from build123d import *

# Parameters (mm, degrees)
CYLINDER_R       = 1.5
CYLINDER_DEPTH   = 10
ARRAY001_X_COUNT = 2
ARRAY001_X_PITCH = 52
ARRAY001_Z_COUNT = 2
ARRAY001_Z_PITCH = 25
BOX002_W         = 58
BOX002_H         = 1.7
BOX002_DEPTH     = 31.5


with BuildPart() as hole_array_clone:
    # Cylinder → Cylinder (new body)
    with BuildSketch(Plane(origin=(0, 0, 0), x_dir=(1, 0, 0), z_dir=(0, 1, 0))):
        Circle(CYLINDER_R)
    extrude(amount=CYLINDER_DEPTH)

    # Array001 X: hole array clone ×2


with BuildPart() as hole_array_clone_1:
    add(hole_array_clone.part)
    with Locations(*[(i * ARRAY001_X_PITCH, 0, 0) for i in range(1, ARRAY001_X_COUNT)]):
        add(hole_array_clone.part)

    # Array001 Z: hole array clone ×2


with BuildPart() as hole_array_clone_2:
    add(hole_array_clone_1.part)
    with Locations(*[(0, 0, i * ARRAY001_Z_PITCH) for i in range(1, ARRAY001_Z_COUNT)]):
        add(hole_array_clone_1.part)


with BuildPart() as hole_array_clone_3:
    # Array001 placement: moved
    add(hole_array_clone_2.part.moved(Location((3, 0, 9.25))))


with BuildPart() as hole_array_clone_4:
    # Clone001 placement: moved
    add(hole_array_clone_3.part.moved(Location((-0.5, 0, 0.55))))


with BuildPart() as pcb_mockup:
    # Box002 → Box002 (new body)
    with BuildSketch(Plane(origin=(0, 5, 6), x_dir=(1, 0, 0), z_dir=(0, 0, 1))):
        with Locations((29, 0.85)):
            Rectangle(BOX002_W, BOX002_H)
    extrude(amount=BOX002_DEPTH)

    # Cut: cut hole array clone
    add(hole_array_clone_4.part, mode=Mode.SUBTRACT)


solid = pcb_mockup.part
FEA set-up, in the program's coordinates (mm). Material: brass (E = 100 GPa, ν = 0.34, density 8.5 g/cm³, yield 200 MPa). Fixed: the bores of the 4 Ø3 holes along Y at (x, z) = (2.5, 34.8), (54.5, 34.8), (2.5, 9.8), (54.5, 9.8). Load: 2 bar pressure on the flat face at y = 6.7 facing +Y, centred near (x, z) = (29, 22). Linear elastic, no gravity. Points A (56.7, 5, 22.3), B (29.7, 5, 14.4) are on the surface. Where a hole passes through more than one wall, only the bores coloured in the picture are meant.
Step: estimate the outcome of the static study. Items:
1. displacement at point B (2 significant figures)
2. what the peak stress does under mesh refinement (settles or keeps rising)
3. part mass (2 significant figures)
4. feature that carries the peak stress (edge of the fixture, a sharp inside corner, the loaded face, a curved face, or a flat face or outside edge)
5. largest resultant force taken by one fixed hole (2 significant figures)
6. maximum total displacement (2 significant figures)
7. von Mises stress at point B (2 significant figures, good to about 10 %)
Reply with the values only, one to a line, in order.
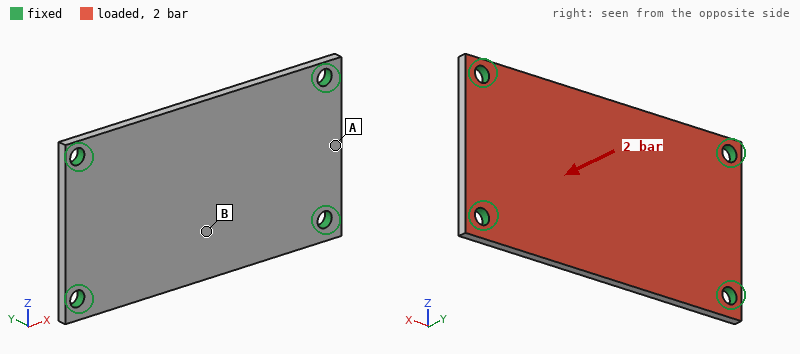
0.100 mm
keeps rising
26 g
edge of the fixture
95 N
0.11 mm
45 MPa
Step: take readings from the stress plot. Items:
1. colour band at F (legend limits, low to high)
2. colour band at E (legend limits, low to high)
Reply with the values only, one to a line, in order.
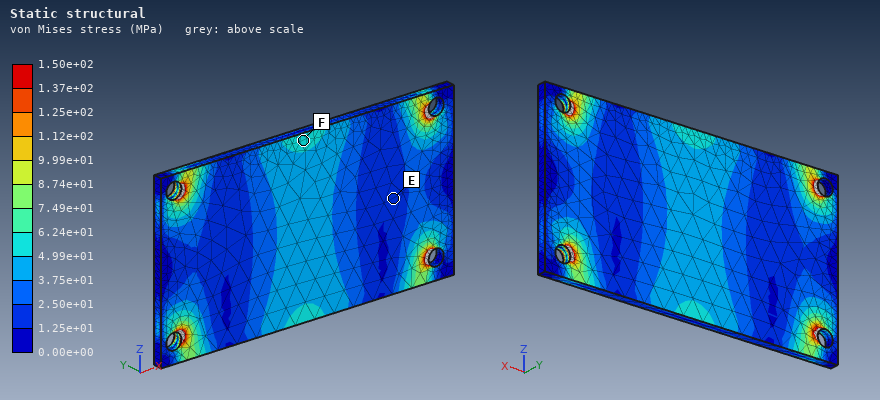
4.99e+01 to 6.24e+01 MPa
1.25e+01 to 2.50e+01 MPa
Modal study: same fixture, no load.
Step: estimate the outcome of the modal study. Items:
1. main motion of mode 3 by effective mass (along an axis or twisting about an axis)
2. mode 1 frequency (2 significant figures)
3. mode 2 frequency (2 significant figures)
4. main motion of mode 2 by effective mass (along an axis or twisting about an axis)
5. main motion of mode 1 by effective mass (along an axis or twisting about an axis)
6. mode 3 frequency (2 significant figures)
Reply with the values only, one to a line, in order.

twisting about Z
2100 Hz
3400 Hz
twisting about X
along Y
5700 Hz
